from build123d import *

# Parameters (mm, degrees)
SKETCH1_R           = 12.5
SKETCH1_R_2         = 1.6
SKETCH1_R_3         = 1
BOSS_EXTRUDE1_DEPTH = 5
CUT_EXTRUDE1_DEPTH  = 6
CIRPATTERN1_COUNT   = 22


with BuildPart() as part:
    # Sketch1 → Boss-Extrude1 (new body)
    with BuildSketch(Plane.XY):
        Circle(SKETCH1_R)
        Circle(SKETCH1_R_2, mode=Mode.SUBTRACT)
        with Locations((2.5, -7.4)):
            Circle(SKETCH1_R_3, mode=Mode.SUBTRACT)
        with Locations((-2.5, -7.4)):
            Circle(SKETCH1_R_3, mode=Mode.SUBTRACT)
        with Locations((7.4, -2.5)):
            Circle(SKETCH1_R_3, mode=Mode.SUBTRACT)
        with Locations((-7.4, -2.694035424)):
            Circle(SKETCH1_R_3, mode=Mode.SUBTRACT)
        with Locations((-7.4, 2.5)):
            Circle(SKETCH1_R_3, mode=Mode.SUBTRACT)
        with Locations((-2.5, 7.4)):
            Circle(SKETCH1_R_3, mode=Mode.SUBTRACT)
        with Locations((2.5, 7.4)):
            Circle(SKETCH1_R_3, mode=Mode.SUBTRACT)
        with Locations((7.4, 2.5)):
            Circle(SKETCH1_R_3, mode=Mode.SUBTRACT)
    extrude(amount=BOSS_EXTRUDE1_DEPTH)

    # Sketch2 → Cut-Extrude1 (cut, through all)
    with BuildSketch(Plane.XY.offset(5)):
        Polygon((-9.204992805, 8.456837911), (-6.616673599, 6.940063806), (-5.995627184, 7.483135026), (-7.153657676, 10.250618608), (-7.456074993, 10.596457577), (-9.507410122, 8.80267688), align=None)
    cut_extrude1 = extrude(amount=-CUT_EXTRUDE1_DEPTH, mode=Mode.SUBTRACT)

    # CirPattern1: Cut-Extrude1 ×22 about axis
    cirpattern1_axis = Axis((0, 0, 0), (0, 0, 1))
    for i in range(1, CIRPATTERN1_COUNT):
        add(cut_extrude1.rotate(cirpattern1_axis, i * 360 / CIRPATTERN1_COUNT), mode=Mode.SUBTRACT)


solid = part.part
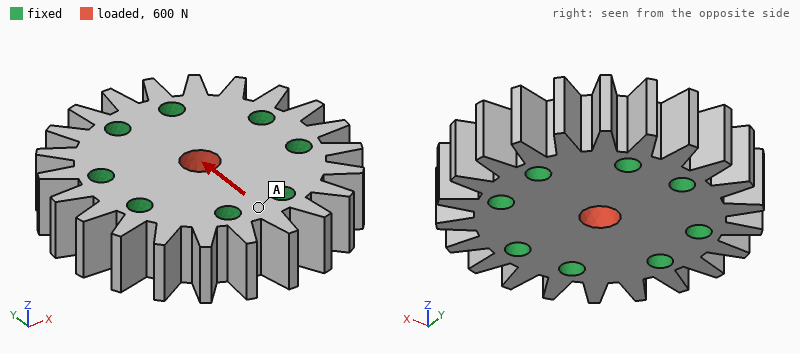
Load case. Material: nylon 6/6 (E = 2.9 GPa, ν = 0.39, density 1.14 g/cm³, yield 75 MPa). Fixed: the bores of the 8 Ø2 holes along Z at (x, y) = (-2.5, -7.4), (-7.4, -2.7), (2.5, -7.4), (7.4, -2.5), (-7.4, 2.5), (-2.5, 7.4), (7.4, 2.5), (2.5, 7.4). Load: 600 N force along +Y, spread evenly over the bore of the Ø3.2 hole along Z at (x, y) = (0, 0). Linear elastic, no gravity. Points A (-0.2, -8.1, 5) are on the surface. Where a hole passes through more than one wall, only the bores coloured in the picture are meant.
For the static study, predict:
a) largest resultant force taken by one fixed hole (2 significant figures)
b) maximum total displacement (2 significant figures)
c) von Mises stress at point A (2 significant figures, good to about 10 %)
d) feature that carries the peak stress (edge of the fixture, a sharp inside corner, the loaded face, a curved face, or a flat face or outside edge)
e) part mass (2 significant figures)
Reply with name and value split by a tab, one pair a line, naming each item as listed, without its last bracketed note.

largest resultant force taken by one fixed hole	130 N
maximum total displacement	17 µm
von Mises stress at point A	2.1 MPa
feature that carries the peak stress	the loaded face
part mass	2.0 g
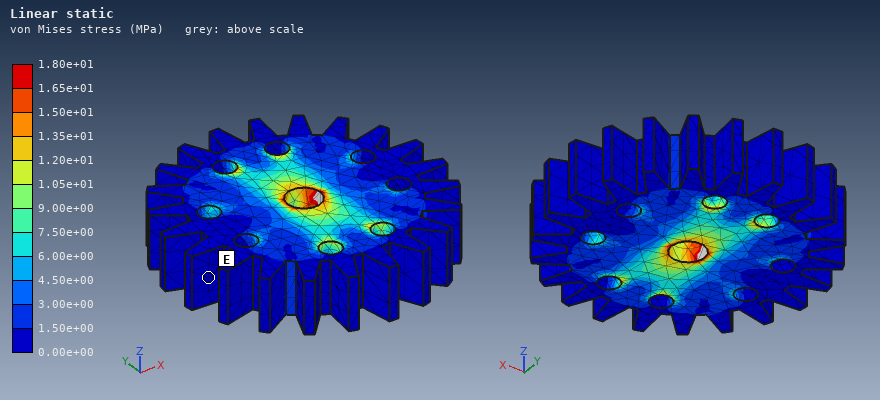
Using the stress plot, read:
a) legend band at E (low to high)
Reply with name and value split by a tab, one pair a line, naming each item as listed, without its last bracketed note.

legend band at E	0.00e+00 to 1.50e+00 MPa
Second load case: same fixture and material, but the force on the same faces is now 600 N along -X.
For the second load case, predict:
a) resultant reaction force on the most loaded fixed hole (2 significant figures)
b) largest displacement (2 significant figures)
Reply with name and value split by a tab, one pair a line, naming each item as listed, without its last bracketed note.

resultant reaction force on the most loaded fixed hole	130 N
largest displacement	17 µm
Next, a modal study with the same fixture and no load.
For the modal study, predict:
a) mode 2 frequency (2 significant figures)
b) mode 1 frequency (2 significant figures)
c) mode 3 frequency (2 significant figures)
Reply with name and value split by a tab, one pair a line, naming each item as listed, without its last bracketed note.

mode 2 frequency	39 kHz
mode 1 frequency	38 kHz
mode 3 frequency	39 kHz
